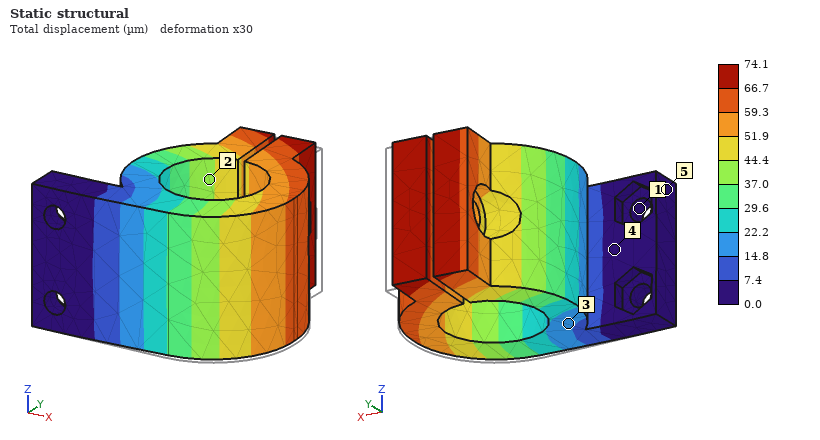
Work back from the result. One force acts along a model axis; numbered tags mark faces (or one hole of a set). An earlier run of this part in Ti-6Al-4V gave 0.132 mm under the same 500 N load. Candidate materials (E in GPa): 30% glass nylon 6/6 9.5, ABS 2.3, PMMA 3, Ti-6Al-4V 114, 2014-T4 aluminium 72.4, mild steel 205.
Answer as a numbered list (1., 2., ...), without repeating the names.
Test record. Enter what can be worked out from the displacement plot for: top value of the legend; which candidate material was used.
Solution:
1. 74.1 µm
2. mild steel
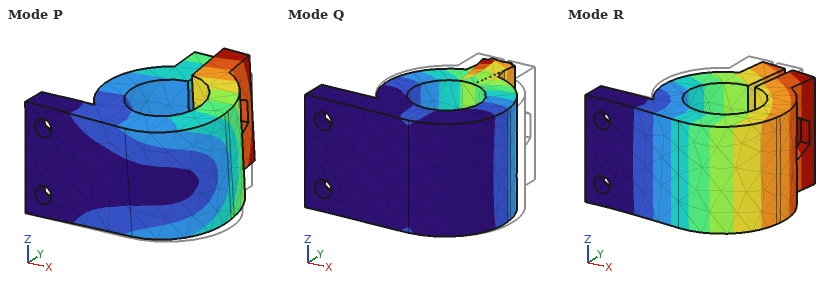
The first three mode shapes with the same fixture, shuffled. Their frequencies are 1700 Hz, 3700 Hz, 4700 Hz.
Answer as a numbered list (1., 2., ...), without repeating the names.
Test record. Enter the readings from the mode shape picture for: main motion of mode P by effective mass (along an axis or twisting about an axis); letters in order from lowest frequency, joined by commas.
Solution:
1. along Z
2. R, P, Q
